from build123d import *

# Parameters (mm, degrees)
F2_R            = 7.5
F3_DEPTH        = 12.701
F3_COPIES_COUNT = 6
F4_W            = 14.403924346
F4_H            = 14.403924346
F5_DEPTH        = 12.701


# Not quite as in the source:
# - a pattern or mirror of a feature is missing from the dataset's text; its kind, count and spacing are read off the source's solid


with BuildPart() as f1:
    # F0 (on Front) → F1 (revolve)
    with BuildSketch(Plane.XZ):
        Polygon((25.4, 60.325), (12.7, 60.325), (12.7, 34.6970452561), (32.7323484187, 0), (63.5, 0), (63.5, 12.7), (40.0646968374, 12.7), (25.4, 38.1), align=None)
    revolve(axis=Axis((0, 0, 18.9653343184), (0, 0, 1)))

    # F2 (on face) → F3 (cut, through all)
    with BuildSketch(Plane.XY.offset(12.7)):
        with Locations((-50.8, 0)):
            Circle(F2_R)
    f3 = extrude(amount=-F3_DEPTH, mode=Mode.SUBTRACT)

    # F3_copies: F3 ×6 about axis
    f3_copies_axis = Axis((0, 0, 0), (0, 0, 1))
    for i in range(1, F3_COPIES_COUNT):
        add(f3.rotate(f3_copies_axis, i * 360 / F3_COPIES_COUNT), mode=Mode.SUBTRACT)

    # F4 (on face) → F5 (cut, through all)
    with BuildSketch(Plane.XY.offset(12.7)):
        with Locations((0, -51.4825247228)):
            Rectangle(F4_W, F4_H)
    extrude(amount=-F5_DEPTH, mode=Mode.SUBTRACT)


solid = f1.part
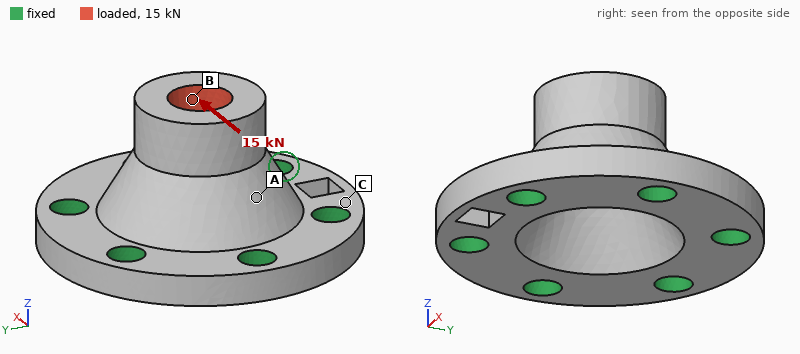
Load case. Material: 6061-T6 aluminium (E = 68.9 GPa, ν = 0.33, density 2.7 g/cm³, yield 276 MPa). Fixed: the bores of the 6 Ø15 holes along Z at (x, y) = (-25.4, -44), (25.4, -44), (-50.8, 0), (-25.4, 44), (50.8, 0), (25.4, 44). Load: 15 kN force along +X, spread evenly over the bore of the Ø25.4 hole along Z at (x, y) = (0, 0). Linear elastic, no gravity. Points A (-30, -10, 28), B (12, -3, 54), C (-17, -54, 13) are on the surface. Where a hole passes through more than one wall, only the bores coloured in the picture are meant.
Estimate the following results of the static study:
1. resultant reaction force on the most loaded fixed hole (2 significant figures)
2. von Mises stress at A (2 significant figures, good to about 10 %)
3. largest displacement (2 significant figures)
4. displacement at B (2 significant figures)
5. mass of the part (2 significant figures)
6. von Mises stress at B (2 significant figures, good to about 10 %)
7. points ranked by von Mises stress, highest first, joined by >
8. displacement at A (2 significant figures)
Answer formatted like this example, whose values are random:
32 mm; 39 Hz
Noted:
6.2 kN; 19 MPa; 32 µm; 28 µm; 550 g; 12 MPa; A > B > C; 12 µm
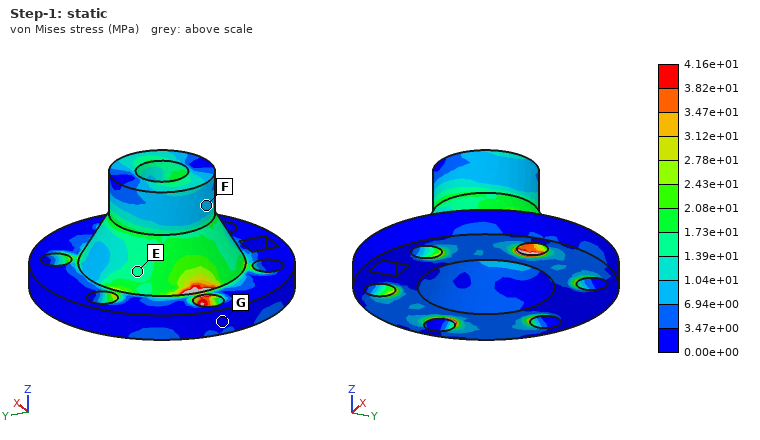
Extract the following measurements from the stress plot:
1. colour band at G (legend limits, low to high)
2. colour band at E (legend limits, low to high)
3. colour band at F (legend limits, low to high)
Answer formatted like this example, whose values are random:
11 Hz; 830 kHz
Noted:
0.00e+00 to 3.47e+00 MPa; 1.39e+01 to 1.73e+01 MPa; 6.94e+00 to 1.04e+01 MPa
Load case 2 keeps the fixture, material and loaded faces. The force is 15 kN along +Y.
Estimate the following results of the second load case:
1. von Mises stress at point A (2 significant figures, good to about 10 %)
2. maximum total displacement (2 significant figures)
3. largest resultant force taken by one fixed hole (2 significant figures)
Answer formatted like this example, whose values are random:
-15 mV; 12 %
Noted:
11 MPa; 32 µm; 5.4 kN
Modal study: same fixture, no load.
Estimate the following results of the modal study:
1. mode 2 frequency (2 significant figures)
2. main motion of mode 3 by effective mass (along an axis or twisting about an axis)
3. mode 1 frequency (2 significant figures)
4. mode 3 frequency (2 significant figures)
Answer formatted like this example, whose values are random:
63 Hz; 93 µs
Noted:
11 kHz; along Z; 11 kHz; 14 kHz
